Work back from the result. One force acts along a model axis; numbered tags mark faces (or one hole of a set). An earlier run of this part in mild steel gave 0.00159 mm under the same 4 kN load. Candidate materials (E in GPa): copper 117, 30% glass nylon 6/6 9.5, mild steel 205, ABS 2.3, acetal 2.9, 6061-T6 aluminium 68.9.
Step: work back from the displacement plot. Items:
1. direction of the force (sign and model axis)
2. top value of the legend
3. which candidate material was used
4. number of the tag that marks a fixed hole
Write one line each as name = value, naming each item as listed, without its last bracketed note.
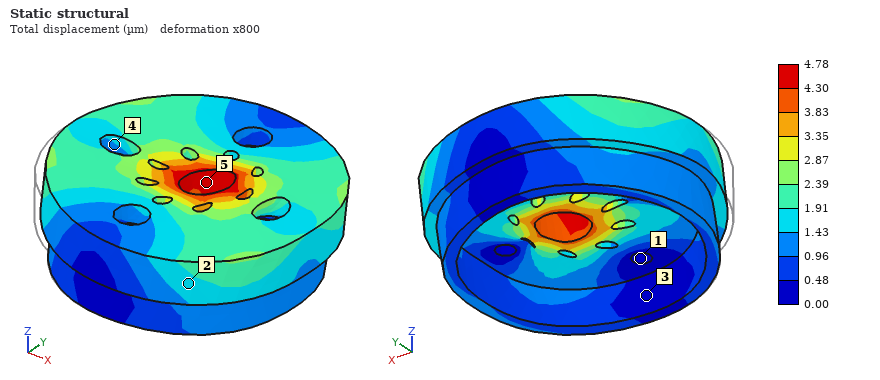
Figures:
direction of the force = +X
top value of the legend = 4.78 µm
which candidate material was used = 6061-T6 aluminium
number of the tag that marks a fixed hole = 1
